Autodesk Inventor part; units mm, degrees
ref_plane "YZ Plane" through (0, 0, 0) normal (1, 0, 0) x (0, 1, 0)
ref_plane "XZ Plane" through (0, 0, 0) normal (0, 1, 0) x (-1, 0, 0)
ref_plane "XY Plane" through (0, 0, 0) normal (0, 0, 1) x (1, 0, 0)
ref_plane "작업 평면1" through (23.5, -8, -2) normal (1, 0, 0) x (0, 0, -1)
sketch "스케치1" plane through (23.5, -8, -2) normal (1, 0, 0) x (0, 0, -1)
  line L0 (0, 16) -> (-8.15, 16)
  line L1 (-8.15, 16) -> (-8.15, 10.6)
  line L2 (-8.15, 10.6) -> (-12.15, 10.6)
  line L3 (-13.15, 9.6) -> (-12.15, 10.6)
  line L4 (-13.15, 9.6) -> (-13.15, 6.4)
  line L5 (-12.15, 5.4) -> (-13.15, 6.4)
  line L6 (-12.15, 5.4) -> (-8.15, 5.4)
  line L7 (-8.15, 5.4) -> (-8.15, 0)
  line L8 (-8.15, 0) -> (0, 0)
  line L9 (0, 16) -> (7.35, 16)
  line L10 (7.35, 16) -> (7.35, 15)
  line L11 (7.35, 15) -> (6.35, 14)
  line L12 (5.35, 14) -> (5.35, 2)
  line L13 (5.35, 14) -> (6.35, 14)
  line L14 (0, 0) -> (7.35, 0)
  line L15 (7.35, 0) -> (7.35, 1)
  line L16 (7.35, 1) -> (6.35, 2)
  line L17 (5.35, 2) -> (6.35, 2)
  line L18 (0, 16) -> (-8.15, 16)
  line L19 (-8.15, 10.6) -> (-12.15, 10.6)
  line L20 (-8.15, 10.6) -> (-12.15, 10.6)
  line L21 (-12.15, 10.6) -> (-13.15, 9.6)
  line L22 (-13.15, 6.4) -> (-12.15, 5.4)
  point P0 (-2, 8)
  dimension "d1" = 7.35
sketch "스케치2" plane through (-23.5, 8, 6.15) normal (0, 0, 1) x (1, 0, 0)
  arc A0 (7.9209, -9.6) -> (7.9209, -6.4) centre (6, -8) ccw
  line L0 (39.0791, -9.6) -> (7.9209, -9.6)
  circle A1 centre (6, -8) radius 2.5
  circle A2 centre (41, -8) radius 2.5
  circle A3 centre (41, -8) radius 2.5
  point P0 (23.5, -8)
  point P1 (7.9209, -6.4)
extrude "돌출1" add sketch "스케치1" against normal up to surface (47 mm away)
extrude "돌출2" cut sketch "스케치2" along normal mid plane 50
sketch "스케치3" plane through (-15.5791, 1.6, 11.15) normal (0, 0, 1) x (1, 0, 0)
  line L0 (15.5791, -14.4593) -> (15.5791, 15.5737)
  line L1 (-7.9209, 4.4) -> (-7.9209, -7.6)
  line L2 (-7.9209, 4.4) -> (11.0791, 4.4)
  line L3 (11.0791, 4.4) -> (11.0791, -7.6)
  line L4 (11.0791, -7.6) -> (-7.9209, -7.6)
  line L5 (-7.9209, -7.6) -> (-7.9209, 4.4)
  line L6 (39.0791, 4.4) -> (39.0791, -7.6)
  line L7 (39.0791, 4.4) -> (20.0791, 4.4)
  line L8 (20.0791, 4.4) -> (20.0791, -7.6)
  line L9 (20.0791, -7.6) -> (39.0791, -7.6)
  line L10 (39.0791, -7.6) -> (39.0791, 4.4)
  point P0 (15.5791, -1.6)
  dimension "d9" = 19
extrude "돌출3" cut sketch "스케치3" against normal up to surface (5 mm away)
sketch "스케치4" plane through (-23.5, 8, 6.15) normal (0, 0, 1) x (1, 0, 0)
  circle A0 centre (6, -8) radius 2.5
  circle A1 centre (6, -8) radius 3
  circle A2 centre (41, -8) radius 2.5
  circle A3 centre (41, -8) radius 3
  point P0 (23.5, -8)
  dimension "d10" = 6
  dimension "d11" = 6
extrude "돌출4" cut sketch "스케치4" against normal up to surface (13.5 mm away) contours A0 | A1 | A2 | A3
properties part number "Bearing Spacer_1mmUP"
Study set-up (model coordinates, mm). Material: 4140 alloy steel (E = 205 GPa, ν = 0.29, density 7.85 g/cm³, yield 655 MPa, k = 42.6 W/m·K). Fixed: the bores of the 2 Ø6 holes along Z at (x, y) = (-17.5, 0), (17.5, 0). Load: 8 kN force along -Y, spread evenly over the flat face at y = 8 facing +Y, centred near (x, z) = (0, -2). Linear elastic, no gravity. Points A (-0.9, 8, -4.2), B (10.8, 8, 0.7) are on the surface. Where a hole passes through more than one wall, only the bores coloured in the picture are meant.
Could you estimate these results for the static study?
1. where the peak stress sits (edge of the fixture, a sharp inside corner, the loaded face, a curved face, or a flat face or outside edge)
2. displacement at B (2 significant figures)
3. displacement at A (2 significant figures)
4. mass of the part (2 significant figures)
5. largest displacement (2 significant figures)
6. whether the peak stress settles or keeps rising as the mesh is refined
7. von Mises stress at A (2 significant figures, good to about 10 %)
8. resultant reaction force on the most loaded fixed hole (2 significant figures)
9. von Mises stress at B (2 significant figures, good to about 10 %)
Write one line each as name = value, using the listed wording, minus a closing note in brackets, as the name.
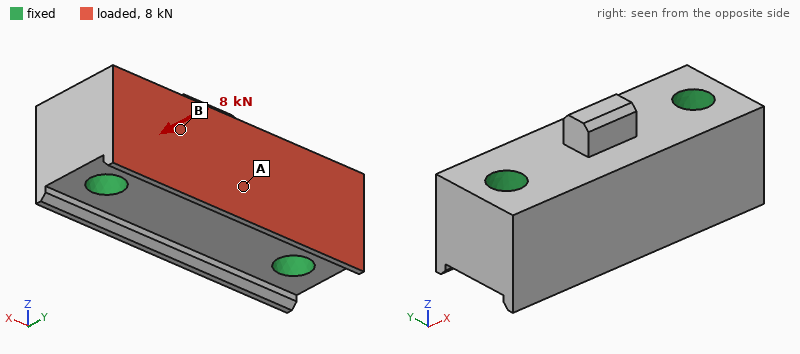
where the peak stress sits = edge of the fixture
displacement at B = 1.6 µm
displacement at A = 2.9 µm
mass of the part = 78 g
largest displacement = 4.6 µm
whether the peak stress settles or keeps rising as the mesh is refined = keeps rising
von Mises stress at A = 29 MPa
resultant reaction force on the most loaded fixed hole = 4.0 kN
von Mises stress at B = 13 MPa
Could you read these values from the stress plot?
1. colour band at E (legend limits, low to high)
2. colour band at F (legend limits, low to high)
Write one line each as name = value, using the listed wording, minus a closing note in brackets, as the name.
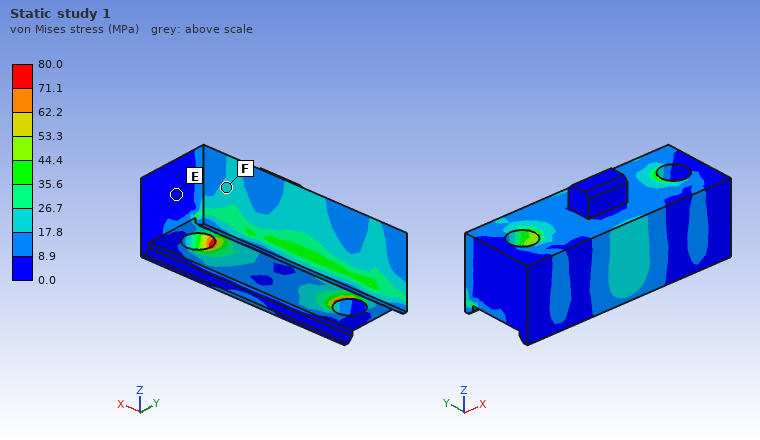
colour band at E = 0.0 to 8.9 MPa
colour band at F = 17.8 to 26.7 MPa
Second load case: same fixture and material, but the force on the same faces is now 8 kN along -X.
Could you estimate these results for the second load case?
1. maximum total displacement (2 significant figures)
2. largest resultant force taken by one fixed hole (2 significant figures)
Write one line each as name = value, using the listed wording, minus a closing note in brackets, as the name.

maximum total displacement = 3.0 µm
largest resultant force taken by one fixed hole = 4.2 kN
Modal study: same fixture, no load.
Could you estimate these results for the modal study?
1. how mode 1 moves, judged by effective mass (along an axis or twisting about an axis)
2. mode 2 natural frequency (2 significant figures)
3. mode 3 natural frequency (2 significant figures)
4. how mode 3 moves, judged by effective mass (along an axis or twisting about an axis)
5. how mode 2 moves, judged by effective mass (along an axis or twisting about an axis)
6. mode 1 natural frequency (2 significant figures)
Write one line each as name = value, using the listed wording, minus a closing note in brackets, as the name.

how mode 1 moves, judged by effective mass = along Y
mode 2 natural frequency = 36 kHz
mode 3 natural frequency = 39 kHz
how mode 3 moves, judged by effective mass = twisting about X
how mode 2 moves, judged by effective mass = along Z
mode 1 natural frequency = 33 kHz
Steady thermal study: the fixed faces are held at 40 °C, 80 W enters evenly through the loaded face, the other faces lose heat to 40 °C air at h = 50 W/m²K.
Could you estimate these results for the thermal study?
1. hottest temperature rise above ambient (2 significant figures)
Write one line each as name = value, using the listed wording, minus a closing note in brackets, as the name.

hottest temperature rise above ambient = 46 K
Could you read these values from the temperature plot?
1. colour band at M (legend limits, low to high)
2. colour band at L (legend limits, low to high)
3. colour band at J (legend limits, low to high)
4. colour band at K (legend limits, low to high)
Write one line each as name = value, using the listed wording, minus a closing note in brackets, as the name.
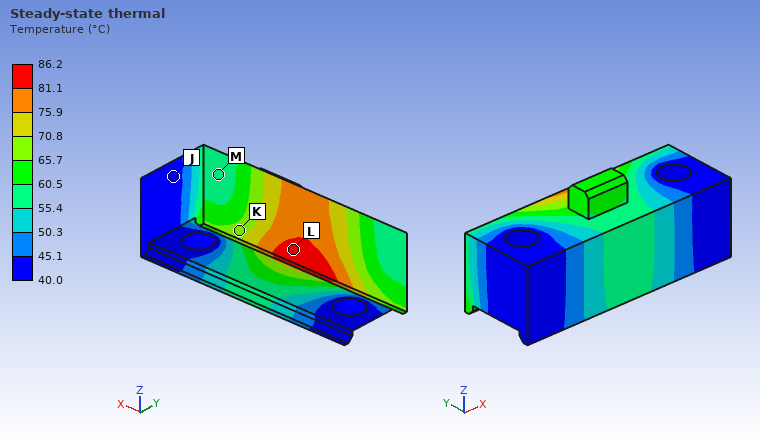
colour band at M = 55.4 to 60.5 °C
colour band at L = 81.1 to 86.2 °C
colour band at J = 40.0 to 45.1 °C
colour band at K = 65.7 to 70.8 °C
